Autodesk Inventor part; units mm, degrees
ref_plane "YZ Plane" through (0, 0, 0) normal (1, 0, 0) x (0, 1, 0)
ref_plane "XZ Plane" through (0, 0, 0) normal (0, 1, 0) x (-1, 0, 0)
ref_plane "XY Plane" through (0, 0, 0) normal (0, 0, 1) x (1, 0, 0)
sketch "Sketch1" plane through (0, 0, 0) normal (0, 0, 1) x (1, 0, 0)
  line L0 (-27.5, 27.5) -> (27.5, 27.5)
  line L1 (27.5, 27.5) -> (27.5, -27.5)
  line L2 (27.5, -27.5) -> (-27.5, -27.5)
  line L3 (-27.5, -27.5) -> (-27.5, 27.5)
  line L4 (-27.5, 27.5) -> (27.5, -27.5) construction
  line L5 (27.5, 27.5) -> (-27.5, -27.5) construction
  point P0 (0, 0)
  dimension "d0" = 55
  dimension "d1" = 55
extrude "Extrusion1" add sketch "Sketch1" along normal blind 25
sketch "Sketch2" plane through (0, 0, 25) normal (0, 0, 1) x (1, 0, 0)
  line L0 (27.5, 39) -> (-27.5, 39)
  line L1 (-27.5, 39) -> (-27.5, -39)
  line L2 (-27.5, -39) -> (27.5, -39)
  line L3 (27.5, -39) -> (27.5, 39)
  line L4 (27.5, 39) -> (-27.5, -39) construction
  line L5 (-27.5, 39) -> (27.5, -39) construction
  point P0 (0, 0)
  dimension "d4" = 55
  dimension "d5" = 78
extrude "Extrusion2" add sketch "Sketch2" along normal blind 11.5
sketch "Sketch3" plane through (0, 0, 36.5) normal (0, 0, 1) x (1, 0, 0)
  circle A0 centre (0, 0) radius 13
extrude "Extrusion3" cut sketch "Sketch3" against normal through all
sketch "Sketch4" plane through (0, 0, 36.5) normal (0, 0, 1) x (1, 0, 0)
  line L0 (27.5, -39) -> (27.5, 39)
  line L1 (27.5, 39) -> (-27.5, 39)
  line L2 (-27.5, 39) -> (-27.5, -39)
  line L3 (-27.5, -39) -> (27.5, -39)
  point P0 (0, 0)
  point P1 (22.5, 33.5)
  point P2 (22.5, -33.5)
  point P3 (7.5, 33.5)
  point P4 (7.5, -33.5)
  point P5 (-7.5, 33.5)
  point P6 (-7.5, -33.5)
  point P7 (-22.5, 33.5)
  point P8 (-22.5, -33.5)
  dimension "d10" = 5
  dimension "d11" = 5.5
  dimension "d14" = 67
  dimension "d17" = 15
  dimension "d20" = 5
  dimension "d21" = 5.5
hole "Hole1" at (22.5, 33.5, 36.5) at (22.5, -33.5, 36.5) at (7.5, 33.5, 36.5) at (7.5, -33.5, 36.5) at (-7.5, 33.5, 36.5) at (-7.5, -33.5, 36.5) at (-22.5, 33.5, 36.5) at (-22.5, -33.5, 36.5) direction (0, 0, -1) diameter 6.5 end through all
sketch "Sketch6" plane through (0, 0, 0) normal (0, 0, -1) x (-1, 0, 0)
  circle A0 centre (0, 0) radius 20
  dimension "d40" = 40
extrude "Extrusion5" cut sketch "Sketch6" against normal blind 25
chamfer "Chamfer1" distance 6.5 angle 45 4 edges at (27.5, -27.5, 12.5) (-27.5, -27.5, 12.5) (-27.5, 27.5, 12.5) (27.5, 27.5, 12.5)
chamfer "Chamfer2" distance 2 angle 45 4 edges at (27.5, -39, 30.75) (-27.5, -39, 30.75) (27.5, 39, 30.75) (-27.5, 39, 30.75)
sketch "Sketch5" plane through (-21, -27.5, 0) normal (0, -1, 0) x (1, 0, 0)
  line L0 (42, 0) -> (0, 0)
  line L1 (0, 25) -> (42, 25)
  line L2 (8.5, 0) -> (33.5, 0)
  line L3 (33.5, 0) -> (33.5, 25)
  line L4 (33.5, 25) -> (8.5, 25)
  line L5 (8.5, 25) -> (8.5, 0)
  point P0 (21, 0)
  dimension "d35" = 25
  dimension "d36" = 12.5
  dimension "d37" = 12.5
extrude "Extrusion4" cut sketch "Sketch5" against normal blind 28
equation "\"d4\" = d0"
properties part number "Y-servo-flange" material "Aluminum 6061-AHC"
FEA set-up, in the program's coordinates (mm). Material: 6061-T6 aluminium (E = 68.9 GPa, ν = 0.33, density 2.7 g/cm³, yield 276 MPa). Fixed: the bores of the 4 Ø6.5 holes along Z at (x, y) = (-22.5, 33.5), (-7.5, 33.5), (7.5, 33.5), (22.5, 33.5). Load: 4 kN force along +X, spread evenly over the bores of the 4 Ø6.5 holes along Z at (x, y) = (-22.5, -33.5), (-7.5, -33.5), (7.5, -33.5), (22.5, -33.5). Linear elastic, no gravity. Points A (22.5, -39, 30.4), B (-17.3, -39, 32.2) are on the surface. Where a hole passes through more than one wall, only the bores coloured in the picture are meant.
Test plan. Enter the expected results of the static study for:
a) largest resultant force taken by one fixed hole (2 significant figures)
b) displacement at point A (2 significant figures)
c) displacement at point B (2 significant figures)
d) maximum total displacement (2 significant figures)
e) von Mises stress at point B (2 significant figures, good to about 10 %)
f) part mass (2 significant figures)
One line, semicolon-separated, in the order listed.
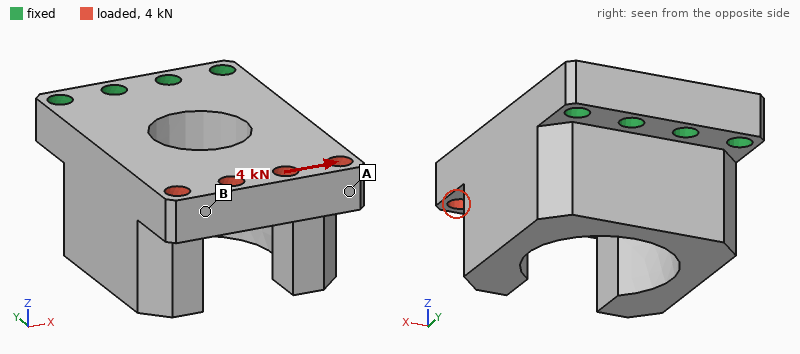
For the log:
5.4 kN; 78 µm; 77 µm; 81 µm; 13 MPa; 210 g
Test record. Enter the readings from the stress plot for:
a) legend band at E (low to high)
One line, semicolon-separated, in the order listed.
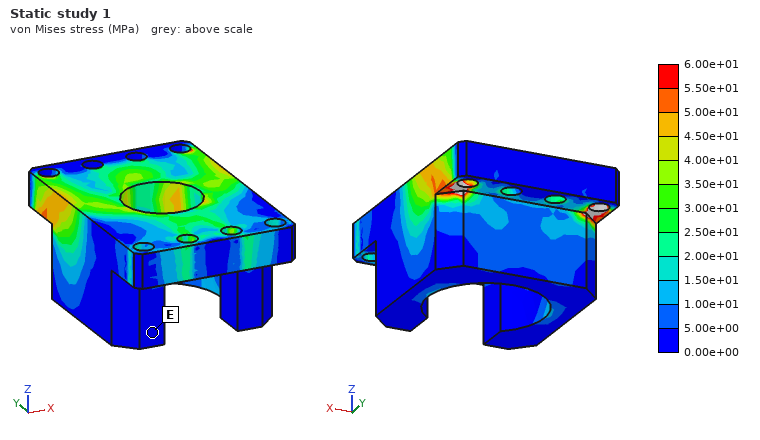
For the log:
0.00e+00 to 5.00e+00 MPa
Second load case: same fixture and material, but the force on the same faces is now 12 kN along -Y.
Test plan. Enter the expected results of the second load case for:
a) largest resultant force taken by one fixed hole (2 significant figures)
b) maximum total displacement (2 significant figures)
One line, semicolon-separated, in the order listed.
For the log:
4.1 kN; 50 µm
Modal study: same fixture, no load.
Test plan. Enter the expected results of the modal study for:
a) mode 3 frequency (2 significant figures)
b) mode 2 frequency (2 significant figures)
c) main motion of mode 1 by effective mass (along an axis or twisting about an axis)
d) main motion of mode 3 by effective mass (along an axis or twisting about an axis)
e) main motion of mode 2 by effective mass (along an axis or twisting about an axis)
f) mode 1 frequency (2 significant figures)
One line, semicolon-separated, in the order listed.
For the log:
4800 Hz; 4500 Hz; along Z; along X; along X; 1900 Hz
